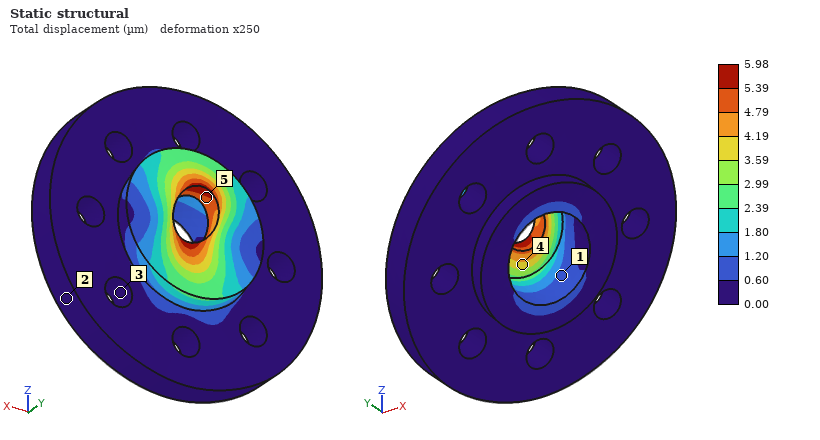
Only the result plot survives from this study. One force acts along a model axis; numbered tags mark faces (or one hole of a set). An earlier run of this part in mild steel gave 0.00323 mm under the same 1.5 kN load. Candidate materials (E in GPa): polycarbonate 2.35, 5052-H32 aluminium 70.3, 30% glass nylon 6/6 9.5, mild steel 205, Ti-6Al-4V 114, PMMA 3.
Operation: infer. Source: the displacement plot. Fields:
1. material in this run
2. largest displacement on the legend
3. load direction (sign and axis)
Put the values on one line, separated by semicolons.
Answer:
Ti-6Al-4V; 5.98 µm; +Z
